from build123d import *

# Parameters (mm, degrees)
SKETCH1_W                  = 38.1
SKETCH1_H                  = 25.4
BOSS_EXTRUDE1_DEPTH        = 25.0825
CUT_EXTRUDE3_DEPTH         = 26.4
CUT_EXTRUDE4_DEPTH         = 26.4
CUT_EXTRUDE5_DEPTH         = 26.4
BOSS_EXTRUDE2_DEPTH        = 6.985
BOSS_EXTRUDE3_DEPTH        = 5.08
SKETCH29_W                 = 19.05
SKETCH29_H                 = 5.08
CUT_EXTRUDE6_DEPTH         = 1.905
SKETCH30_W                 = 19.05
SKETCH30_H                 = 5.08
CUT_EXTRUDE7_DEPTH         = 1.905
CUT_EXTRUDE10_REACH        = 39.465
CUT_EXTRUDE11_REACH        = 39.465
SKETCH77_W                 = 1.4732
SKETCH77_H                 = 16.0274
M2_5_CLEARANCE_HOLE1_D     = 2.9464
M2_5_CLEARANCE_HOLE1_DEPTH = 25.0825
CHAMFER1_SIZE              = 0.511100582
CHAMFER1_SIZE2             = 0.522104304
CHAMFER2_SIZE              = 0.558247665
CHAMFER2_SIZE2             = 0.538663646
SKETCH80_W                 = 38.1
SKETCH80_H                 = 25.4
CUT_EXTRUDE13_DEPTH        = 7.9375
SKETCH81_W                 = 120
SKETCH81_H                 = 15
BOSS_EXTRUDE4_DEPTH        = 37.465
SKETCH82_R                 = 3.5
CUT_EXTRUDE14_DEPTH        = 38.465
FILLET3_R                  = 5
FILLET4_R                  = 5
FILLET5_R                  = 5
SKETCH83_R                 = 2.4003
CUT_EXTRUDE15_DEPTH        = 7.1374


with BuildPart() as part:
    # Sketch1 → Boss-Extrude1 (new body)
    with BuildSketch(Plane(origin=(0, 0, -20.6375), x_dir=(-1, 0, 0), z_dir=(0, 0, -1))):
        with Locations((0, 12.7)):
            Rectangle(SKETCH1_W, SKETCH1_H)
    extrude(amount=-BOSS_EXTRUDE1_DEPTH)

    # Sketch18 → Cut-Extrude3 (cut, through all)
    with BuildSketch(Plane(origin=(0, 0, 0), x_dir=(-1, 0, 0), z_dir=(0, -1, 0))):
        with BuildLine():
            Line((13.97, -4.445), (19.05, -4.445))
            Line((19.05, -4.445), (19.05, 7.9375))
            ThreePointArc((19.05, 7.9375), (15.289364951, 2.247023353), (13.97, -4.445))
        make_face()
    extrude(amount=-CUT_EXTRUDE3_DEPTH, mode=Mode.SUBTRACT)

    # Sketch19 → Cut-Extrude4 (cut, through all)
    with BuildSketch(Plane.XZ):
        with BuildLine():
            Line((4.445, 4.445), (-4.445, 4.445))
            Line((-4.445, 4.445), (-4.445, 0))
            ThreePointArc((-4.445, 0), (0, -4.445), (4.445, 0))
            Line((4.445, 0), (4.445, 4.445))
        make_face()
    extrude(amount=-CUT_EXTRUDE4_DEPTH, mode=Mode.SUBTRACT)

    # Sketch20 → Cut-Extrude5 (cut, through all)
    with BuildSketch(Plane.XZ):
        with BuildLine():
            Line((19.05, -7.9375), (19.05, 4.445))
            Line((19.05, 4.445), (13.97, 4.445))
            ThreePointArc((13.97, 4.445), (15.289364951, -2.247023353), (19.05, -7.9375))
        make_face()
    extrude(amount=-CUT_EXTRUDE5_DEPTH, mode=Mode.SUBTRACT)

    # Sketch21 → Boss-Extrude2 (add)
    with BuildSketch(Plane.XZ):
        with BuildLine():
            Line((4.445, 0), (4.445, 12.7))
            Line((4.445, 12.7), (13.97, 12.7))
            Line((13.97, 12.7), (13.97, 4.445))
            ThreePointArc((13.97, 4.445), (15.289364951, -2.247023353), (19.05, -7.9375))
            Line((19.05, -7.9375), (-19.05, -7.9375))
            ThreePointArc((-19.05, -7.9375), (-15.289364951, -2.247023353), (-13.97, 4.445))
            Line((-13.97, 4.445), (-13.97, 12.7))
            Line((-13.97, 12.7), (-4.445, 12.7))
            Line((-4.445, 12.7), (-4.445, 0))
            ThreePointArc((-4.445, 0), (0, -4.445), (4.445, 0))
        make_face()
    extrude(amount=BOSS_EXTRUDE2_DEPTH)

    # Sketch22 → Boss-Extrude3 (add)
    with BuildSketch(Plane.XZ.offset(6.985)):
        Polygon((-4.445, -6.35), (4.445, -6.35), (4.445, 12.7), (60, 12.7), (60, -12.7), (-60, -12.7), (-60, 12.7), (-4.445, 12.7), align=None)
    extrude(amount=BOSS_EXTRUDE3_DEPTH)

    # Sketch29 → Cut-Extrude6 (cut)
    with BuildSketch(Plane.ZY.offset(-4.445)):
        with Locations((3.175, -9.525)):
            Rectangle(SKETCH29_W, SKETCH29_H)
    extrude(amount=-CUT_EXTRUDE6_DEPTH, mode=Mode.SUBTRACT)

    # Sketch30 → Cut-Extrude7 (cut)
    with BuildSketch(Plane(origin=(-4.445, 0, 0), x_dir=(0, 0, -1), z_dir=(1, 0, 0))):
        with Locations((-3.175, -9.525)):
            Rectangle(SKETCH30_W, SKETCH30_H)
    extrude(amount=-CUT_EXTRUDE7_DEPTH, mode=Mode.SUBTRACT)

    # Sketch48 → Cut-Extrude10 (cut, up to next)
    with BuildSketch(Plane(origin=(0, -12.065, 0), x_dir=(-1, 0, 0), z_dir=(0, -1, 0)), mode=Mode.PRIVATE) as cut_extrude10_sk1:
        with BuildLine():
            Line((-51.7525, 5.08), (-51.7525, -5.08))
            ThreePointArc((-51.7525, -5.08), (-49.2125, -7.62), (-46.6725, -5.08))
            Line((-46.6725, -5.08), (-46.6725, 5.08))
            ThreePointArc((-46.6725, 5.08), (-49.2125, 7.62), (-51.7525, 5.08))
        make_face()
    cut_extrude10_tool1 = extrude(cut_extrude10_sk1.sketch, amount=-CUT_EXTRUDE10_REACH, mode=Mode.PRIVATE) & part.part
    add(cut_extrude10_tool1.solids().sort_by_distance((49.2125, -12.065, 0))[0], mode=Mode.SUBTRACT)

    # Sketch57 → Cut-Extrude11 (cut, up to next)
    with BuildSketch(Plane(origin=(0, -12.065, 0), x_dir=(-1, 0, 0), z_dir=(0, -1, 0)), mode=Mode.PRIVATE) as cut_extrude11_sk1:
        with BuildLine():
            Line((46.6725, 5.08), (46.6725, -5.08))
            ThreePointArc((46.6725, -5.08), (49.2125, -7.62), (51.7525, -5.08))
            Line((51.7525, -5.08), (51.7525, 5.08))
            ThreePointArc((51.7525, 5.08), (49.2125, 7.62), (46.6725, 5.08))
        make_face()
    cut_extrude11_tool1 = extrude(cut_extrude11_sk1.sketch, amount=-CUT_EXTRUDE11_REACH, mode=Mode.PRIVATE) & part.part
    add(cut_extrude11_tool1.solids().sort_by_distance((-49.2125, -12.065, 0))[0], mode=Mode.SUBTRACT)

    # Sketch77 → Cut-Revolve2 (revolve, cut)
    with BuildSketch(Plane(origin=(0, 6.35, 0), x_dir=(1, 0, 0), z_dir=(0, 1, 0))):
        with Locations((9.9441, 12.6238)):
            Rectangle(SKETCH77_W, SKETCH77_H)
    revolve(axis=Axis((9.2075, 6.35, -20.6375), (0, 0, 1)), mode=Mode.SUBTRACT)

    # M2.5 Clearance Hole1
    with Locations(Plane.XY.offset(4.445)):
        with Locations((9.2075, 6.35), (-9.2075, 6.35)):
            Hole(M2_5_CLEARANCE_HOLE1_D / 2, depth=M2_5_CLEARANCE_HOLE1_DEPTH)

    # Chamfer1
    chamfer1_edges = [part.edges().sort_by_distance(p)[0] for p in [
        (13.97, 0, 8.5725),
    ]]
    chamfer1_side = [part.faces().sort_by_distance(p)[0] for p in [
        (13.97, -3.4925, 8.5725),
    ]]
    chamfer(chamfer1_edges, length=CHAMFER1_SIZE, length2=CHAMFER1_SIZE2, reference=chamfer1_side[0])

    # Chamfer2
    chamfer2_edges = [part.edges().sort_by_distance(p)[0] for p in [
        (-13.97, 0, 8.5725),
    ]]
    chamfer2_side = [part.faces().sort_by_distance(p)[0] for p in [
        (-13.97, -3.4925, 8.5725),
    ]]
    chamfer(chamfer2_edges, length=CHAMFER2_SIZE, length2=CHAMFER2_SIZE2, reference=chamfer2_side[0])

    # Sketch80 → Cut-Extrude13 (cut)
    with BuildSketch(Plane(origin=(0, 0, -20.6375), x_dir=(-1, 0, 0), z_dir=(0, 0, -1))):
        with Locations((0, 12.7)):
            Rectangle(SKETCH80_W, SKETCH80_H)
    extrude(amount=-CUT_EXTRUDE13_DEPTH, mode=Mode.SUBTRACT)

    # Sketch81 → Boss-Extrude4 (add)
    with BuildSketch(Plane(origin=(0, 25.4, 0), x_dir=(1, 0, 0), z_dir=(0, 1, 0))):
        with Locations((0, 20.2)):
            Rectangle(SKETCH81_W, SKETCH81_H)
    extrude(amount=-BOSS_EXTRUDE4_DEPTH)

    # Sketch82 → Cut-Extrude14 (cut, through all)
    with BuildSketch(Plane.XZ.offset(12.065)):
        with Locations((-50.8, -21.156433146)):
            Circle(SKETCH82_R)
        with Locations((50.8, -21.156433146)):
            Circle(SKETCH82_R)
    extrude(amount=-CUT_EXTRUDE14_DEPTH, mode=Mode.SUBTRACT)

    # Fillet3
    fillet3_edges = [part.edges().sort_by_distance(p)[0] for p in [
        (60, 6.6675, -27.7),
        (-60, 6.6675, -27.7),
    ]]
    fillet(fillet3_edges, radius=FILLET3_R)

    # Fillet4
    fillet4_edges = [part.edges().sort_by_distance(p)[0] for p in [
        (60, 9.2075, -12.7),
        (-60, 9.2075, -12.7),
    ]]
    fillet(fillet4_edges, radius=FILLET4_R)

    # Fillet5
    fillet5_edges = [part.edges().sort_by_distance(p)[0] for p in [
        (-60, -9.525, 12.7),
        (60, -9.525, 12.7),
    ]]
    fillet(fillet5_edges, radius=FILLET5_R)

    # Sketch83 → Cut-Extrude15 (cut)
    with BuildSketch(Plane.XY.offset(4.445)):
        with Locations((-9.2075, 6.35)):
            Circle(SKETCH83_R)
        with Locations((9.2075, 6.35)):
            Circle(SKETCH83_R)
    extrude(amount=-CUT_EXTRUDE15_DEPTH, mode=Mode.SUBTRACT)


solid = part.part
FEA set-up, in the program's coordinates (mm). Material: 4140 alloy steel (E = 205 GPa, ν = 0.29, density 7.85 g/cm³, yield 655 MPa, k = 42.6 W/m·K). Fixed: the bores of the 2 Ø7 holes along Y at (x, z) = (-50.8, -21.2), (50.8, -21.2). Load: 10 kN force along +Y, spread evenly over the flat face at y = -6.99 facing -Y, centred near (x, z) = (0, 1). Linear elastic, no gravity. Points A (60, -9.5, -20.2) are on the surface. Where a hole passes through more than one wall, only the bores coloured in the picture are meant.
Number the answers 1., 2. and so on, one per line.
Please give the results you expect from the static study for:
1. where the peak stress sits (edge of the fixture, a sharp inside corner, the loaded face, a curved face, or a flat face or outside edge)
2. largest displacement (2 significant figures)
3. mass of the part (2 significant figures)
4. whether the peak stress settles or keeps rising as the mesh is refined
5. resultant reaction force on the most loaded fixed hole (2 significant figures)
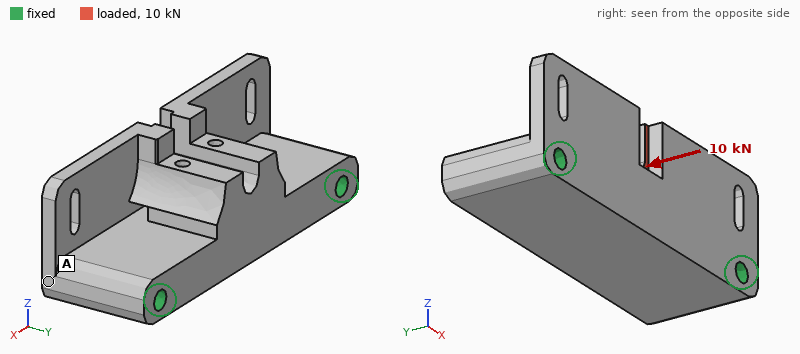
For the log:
1. edge of the fixture
2. 54 µm
3. 730 g
4. keeps rising
5. 5.0 kN
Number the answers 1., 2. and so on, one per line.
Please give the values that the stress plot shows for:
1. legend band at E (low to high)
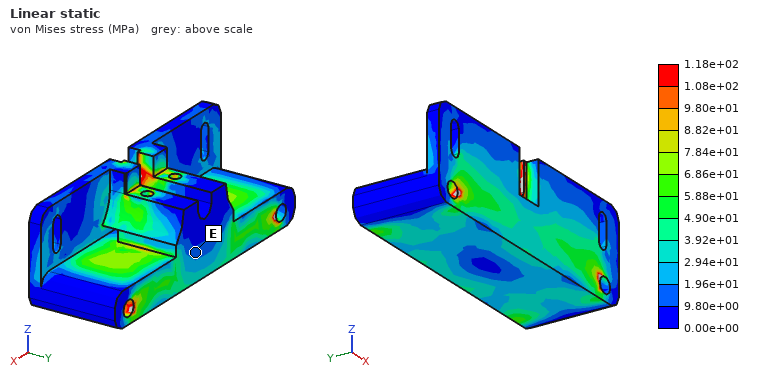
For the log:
1. 9.80e+00 to 1.96e+01 MPa
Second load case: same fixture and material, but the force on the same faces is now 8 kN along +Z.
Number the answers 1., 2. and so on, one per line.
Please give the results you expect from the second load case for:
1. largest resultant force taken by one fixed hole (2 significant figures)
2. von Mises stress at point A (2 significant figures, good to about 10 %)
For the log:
1. 4.9 kN
2. 13 MPa
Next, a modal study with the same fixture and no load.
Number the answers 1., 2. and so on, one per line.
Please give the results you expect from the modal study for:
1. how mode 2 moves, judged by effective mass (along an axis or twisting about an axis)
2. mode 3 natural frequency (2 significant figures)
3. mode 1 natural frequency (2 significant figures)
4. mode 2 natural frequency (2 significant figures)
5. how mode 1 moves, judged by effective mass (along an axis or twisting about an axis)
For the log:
1. along Z
2. 6900 Hz
3. 5800 Hz
4. 6300 Hz
5. along Y
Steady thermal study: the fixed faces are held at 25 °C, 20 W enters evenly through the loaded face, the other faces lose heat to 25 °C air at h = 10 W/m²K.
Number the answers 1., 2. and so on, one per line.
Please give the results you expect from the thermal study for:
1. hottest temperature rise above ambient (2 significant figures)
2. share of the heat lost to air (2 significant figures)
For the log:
1. 34 K
2. 9.6 %
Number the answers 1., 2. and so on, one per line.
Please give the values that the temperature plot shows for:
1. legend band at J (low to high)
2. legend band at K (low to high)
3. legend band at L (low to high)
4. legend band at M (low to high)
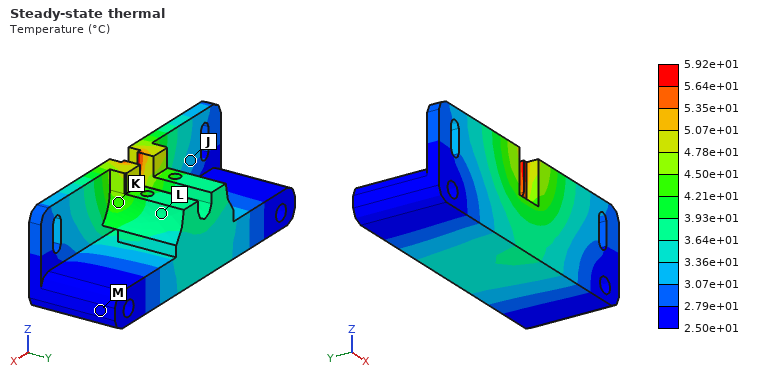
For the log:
1. 3.07e+01 to 3.36e+01 °C
2. 4.21e+01 to 4.50e+01 °C
3. 3.64e+01 to 3.93e+01 °C
4. 2.50e+01 to 2.79e+01 °C
